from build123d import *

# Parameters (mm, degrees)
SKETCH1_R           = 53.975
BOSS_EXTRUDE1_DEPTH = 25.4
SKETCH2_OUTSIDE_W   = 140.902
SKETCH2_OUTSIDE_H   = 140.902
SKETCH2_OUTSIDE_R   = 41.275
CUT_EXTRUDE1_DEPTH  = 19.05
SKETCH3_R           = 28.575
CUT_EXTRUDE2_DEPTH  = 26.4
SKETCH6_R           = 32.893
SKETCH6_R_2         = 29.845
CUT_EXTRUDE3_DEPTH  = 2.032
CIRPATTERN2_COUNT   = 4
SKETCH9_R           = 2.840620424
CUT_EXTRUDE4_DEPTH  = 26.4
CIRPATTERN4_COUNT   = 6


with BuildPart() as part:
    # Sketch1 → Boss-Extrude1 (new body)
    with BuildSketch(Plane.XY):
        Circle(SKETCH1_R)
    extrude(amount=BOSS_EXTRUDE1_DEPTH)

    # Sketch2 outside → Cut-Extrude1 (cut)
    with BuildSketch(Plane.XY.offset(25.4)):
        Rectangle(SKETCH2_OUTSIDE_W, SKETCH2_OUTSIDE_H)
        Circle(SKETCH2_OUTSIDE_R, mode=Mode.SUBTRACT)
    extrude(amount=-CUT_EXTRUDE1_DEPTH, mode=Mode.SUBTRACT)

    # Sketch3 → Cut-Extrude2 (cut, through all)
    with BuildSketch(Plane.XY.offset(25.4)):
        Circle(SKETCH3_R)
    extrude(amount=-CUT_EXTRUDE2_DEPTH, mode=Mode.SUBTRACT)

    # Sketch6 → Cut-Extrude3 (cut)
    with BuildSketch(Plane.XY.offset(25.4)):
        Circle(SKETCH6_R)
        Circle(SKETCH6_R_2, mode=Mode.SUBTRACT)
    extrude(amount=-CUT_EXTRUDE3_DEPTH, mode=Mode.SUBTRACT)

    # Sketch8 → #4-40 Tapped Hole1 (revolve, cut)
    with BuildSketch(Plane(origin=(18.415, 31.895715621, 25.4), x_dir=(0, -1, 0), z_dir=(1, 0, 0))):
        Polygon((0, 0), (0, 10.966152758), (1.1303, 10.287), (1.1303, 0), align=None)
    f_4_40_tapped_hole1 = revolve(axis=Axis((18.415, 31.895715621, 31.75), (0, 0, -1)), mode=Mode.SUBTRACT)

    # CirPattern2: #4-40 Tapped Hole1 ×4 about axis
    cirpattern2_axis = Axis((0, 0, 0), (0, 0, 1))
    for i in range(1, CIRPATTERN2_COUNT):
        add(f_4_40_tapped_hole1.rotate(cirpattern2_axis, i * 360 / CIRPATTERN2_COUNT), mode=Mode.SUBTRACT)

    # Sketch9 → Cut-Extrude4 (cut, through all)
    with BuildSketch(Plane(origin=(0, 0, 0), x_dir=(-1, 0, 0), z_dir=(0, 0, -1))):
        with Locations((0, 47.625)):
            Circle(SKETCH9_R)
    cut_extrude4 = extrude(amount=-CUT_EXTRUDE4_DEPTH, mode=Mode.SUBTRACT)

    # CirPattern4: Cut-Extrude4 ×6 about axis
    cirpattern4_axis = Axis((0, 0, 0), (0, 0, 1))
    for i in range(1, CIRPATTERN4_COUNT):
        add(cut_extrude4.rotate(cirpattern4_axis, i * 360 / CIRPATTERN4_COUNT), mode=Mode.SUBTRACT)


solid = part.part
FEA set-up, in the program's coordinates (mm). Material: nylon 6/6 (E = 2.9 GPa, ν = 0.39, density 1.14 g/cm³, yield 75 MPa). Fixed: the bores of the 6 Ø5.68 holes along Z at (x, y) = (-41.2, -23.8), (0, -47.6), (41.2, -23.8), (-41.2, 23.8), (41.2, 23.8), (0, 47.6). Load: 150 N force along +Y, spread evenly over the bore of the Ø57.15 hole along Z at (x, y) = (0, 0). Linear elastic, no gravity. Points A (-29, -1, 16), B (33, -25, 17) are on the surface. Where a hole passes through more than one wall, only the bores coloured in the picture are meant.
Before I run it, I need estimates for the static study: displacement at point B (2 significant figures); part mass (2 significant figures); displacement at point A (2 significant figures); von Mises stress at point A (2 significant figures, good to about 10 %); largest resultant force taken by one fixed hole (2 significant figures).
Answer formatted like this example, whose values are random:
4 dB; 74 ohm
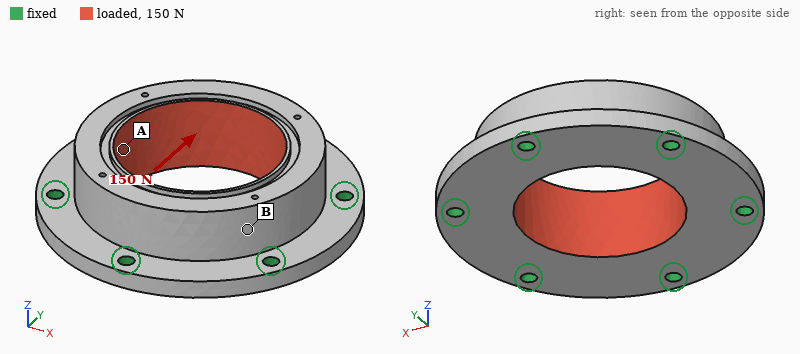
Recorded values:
1.9 µm; 110 g; 1.8 µm; 0.13 MPa; 30 N
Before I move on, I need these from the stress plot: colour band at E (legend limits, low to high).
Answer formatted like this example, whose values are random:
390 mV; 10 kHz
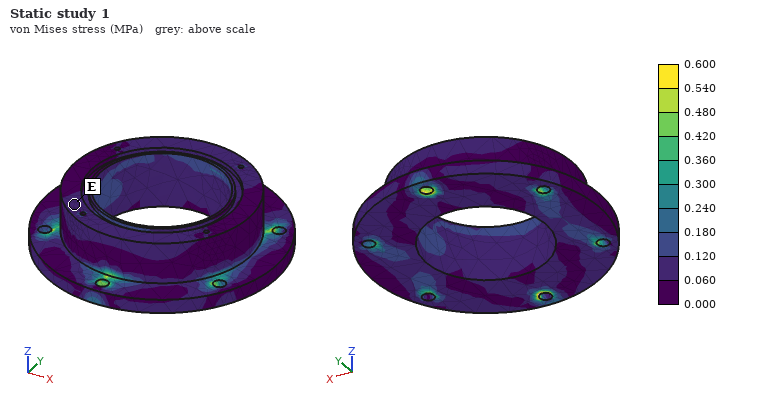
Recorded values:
0.060 to 0.120 MPa
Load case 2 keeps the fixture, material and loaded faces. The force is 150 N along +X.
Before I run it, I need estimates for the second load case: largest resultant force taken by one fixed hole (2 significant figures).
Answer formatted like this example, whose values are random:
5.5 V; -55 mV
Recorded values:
28 N
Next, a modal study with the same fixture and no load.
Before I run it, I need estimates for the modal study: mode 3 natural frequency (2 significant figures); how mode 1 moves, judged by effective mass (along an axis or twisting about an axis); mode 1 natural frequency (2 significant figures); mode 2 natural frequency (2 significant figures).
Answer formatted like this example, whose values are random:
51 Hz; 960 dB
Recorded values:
4000 Hz; along Z; 3500 Hz; 4000 Hz
